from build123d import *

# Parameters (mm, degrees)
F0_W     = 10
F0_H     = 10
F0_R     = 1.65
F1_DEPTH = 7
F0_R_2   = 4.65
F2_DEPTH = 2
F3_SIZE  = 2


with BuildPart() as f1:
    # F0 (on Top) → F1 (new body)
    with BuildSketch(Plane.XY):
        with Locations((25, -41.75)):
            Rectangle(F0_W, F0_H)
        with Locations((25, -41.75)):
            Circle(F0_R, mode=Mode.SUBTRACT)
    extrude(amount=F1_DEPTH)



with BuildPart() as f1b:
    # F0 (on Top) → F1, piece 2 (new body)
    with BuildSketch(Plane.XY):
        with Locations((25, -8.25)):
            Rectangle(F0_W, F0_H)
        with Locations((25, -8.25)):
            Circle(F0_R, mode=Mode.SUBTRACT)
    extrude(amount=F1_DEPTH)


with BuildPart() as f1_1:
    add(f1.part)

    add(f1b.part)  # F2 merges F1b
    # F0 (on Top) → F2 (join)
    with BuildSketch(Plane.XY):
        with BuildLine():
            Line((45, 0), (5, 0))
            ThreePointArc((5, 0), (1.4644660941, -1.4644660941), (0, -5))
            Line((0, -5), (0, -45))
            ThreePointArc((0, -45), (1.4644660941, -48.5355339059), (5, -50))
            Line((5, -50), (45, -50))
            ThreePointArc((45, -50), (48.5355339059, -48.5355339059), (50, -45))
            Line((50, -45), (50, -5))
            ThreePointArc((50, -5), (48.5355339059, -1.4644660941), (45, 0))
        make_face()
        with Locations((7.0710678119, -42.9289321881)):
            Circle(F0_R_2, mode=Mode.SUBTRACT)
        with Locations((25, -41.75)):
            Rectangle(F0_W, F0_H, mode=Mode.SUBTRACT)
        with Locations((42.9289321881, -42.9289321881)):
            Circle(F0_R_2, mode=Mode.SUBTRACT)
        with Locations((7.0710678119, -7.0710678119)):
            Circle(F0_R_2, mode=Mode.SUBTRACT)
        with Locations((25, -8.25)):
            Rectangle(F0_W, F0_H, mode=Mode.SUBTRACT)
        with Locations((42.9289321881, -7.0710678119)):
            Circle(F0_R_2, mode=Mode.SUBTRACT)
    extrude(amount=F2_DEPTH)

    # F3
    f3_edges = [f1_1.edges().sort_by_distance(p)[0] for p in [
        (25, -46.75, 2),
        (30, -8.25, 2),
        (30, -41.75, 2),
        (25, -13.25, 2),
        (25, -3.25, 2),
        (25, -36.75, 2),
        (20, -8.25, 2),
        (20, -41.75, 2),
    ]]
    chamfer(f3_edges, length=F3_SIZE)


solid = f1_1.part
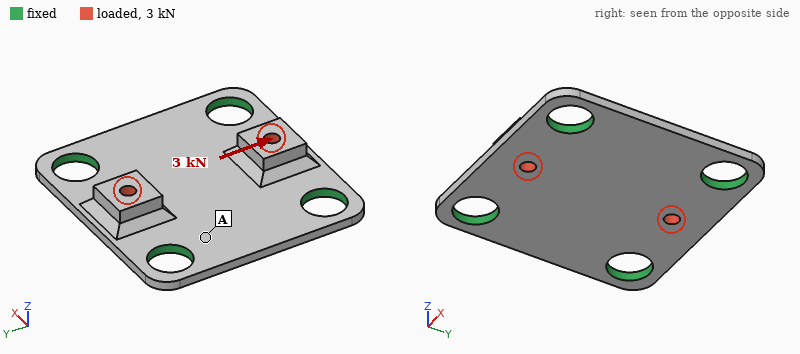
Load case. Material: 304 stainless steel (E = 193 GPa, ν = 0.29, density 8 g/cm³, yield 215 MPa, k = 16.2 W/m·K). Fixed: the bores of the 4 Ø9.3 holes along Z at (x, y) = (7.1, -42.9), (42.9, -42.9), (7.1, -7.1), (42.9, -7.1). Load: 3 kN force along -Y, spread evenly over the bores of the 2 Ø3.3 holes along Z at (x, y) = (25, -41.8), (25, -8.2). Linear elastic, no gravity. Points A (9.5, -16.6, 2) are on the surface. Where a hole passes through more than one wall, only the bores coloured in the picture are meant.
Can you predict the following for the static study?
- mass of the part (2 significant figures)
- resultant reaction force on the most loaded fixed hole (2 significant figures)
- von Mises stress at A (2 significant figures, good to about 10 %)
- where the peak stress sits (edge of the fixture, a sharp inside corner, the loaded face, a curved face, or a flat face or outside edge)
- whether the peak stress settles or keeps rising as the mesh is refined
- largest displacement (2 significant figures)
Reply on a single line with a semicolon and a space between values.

44 g; 810 N; 16 MPa; edge of the fixture; keeps rising; 14 µm
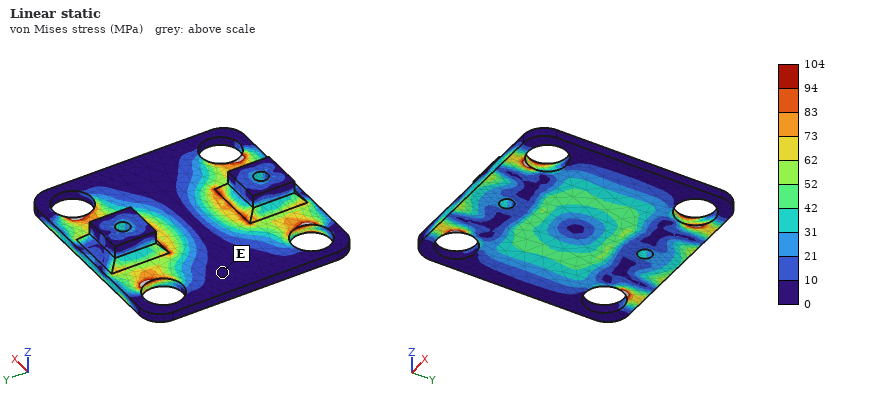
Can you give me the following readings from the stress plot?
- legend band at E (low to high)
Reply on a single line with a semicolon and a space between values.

0 to 10 MPa
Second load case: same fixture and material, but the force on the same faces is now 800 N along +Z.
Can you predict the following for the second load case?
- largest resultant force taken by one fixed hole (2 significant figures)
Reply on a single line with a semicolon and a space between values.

250 N
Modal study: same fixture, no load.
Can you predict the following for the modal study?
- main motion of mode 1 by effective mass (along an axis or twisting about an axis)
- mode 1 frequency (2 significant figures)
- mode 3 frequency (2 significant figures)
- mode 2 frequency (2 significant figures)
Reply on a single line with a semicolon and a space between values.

along Z; 8600 Hz; 13 kHz; 13 kHz
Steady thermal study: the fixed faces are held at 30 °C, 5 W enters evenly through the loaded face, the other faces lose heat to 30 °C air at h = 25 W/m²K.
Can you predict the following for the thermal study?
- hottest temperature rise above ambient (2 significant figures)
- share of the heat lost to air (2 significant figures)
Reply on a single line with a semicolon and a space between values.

24 K; 21 %
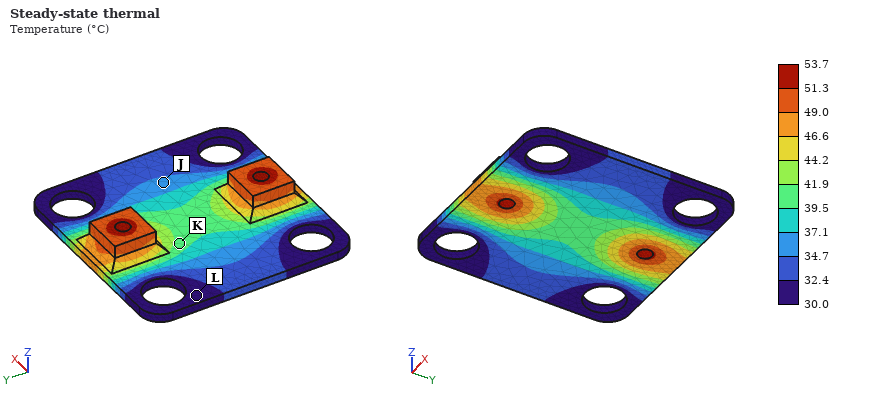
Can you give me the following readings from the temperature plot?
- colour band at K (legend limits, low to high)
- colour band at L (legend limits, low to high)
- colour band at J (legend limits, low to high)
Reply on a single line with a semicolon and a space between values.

39.5 to 41.9 °C; 30.0 to 32.4 °C; 34.7 to 37.1 °C
